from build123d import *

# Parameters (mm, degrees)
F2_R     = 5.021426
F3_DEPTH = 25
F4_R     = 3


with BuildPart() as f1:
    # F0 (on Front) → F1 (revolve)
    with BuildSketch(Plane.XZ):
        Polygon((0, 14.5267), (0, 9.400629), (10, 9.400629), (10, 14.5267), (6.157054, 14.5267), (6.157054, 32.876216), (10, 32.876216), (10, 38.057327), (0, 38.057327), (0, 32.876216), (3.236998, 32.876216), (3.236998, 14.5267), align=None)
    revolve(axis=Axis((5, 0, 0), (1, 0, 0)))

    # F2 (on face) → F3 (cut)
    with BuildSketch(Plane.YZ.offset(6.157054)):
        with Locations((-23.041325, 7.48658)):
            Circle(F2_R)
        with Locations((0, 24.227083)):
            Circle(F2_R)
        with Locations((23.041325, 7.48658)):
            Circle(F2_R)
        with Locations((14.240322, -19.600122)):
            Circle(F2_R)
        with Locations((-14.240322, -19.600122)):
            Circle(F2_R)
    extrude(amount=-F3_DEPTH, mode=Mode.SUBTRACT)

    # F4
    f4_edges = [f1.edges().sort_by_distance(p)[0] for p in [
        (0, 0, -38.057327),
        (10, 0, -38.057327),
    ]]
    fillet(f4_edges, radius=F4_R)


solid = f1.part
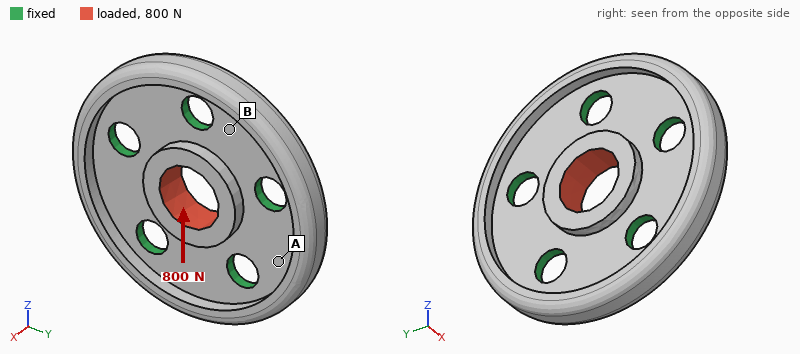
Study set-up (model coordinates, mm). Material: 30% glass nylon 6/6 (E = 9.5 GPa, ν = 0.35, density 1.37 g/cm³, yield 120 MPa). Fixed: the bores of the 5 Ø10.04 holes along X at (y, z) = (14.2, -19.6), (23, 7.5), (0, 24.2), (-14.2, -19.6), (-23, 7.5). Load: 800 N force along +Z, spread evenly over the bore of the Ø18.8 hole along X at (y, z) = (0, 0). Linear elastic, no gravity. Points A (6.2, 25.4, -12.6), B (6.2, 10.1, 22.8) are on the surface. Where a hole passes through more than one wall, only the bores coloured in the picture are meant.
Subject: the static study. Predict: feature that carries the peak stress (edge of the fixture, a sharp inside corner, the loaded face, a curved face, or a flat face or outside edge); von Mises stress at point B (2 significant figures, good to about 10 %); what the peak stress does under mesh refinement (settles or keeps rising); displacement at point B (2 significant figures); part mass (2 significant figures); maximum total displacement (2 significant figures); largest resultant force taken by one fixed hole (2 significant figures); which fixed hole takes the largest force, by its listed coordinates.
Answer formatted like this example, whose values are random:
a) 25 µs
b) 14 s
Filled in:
a) edge of the fixture
b) 1.2 MPa
c) keeps rising
d) 1.4 µm
e) 29 g
f) 6.0 µm
g) 230 N
h) (0, 24.2)
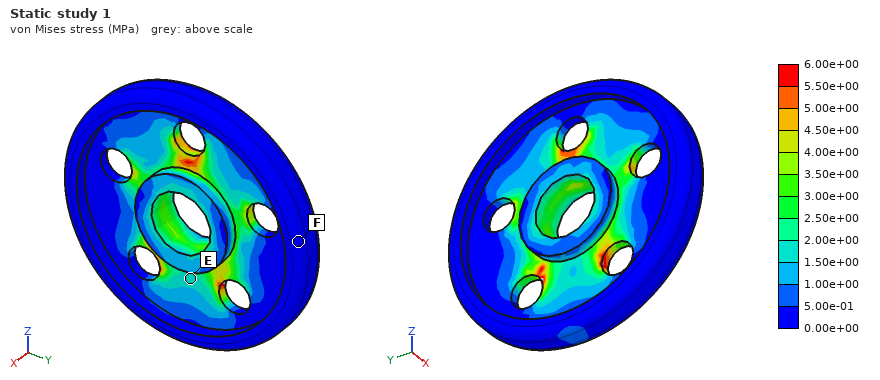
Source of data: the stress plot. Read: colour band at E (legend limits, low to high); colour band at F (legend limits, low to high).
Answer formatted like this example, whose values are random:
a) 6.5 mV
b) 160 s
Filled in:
a) 1.50e+00 to 2.00e+00 MPa
b) 0.00e+00 to 5.00e-01 MPa
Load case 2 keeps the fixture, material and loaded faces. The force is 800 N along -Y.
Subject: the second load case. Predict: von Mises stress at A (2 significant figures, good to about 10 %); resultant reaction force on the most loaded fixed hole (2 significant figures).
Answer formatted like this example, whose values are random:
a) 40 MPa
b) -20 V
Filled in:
a) 0.93 MPa
b) 220 N
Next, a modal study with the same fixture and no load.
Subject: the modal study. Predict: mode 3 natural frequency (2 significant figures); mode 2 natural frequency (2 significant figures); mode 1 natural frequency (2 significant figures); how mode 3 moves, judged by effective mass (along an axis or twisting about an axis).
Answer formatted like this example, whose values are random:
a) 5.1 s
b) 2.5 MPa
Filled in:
a) 6100 Hz
b) 5400 Hz
c) 5400 Hz
d) twisting about Z
